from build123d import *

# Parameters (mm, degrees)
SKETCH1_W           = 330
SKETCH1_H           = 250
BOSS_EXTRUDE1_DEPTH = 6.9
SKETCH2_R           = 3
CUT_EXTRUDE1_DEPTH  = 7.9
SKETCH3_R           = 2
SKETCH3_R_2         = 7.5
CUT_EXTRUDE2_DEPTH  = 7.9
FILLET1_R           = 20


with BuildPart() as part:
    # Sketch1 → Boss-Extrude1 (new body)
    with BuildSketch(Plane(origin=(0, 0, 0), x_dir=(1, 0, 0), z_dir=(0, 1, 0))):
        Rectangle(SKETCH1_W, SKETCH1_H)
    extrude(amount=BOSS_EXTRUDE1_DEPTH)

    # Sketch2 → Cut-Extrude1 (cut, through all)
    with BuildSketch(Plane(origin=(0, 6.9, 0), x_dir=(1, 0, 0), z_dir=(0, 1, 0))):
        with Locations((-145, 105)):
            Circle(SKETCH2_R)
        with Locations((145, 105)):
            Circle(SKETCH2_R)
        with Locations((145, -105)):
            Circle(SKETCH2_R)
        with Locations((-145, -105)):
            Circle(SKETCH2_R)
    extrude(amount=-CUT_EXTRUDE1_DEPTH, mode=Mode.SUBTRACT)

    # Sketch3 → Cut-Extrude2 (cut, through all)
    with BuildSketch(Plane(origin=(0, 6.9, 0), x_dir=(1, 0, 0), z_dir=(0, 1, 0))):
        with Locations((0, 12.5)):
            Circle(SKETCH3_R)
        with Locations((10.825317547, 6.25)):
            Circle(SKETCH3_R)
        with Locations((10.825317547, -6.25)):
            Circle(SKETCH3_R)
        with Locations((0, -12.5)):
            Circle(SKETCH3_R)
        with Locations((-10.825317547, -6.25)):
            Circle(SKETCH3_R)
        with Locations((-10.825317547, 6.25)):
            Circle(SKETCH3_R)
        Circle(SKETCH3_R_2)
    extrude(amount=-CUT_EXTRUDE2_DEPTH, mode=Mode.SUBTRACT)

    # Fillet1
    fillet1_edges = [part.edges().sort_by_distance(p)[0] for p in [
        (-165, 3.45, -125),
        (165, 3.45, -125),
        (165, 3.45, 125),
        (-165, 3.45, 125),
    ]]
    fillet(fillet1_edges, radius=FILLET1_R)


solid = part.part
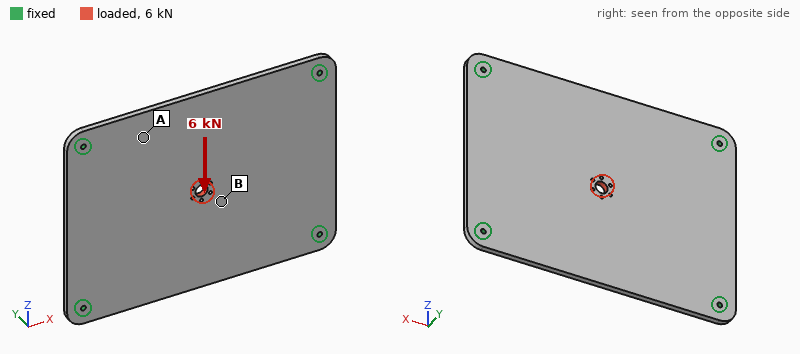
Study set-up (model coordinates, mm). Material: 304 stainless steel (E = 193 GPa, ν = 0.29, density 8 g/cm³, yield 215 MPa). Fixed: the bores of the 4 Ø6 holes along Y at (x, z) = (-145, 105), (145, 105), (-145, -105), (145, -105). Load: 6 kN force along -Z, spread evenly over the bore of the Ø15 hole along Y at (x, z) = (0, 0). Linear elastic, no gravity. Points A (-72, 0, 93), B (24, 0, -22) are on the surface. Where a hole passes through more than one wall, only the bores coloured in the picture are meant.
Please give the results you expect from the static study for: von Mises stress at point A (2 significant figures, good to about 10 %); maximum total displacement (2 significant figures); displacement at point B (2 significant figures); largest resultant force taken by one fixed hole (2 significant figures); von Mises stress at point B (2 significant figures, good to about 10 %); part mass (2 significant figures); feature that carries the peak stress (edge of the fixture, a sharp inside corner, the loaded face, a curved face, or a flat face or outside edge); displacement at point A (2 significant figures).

2.5 MPa
7.6 µm
5.1 µm
1.8 kN
6.2 MPa
4.5 kg
a curved face
3.3 µm
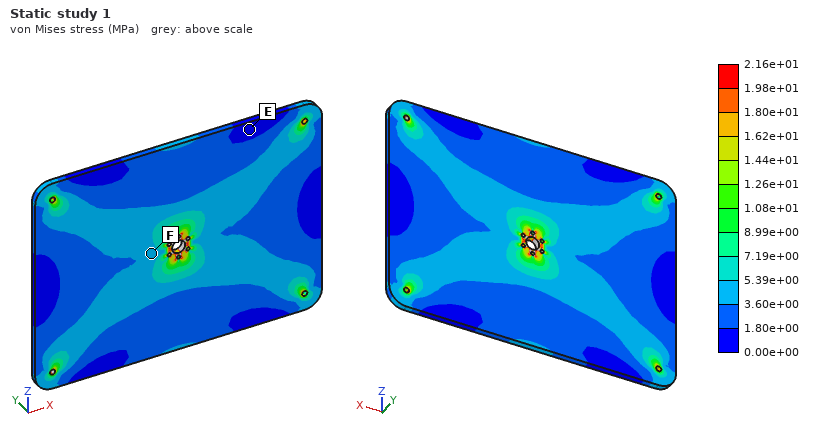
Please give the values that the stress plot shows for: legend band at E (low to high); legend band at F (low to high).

0.00e+00 to 1.80e+00 MPa
3.60e+00 to 5.39e+00 MPa
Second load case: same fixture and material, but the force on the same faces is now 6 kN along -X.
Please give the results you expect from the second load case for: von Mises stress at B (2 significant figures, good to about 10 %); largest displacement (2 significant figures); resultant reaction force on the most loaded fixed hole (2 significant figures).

6.1 MPa
5.9 µm
1.6 kN
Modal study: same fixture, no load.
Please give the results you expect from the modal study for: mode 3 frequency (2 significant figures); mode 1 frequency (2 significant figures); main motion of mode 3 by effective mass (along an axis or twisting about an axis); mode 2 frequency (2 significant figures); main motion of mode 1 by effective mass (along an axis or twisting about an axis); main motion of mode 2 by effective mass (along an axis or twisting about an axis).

690 Hz
300 Hz
twisting about Z
490 Hz
along Y
twisting about X
